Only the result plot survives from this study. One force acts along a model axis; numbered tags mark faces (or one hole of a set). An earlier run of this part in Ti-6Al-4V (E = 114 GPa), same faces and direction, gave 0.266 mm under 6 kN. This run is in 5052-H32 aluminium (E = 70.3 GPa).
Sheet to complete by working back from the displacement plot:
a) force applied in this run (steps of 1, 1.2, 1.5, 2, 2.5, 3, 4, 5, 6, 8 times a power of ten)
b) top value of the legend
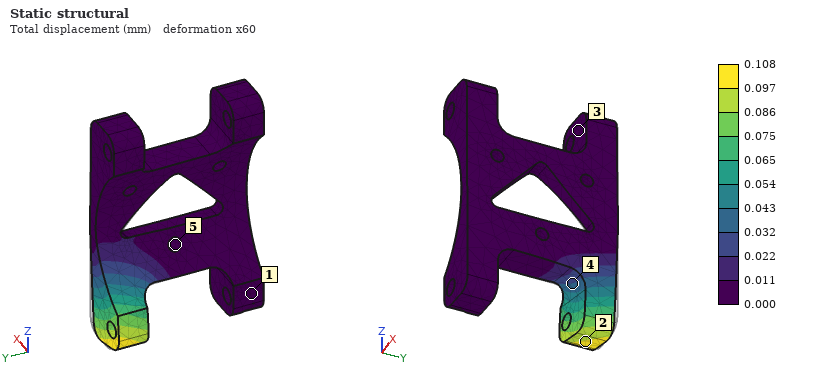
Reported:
1.5 kN
0.108 mm
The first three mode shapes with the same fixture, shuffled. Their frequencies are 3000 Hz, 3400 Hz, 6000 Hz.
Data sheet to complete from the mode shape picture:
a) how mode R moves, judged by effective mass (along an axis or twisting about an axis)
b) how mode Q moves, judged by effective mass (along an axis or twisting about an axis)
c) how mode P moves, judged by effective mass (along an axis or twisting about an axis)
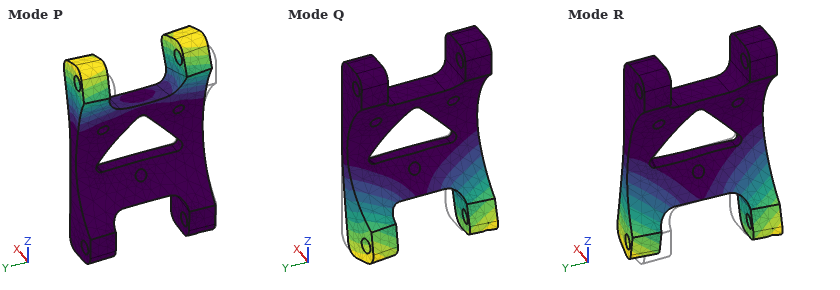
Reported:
twisting about Z
along X
along X
